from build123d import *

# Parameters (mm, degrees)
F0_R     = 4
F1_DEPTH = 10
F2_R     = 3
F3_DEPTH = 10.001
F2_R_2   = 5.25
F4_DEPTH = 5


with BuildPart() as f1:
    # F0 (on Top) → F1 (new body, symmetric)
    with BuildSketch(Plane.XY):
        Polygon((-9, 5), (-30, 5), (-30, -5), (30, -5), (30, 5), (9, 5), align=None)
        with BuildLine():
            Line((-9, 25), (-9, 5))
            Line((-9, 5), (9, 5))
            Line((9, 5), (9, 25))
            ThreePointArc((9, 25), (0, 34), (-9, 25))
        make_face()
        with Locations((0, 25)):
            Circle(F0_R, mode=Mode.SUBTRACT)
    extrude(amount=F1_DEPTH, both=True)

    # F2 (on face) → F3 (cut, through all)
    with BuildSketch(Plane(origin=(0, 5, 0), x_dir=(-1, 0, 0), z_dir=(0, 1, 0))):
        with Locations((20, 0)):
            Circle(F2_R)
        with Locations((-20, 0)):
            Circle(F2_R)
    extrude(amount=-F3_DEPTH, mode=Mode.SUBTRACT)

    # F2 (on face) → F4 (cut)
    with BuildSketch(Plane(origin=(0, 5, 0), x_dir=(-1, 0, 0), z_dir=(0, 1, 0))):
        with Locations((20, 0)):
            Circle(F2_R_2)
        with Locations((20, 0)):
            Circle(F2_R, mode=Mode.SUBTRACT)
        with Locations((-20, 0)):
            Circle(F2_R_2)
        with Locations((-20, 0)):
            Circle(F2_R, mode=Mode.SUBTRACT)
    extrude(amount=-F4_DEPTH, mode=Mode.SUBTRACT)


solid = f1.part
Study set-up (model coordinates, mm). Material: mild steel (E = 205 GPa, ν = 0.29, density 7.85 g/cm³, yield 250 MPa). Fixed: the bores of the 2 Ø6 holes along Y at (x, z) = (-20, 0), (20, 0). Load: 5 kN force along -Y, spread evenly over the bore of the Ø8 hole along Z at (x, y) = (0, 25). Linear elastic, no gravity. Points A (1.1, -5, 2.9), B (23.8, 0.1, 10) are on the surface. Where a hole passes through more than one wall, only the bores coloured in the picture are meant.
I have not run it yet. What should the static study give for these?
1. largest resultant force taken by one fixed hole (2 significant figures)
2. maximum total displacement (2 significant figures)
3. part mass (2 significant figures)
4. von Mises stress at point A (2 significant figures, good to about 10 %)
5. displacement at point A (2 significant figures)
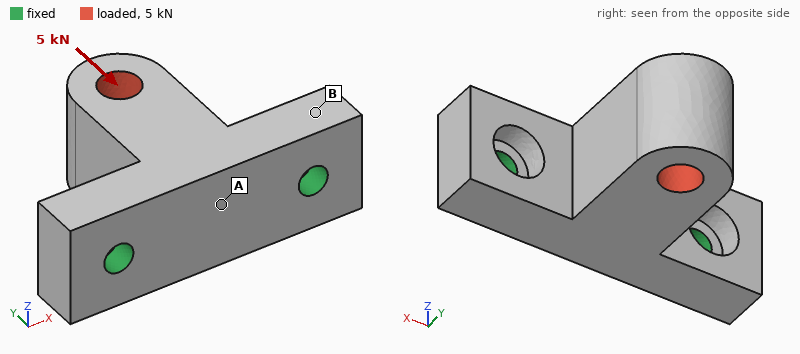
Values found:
3.0 kN
8.6 µm
150 g
26 MPa
6.3 µm
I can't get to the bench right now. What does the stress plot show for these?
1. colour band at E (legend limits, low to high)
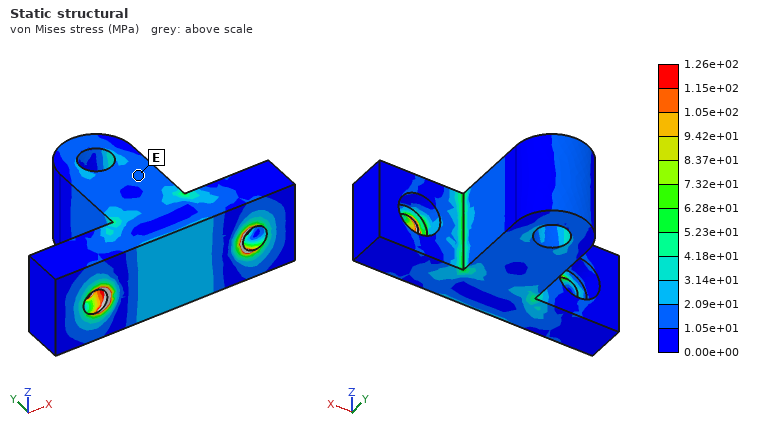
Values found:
1.05e+01 to 2.09e+01 MPa
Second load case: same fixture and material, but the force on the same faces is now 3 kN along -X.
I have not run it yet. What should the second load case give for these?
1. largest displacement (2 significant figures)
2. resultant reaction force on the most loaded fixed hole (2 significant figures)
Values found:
24 µm
2.8 kN
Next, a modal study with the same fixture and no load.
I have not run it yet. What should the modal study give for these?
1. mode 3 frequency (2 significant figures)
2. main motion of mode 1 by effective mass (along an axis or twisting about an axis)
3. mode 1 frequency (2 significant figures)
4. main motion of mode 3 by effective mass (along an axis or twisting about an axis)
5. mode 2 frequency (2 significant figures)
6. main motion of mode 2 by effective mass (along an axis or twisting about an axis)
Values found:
13 kHz
along Z
4500 Hz
along Y
10 kHz
along X
